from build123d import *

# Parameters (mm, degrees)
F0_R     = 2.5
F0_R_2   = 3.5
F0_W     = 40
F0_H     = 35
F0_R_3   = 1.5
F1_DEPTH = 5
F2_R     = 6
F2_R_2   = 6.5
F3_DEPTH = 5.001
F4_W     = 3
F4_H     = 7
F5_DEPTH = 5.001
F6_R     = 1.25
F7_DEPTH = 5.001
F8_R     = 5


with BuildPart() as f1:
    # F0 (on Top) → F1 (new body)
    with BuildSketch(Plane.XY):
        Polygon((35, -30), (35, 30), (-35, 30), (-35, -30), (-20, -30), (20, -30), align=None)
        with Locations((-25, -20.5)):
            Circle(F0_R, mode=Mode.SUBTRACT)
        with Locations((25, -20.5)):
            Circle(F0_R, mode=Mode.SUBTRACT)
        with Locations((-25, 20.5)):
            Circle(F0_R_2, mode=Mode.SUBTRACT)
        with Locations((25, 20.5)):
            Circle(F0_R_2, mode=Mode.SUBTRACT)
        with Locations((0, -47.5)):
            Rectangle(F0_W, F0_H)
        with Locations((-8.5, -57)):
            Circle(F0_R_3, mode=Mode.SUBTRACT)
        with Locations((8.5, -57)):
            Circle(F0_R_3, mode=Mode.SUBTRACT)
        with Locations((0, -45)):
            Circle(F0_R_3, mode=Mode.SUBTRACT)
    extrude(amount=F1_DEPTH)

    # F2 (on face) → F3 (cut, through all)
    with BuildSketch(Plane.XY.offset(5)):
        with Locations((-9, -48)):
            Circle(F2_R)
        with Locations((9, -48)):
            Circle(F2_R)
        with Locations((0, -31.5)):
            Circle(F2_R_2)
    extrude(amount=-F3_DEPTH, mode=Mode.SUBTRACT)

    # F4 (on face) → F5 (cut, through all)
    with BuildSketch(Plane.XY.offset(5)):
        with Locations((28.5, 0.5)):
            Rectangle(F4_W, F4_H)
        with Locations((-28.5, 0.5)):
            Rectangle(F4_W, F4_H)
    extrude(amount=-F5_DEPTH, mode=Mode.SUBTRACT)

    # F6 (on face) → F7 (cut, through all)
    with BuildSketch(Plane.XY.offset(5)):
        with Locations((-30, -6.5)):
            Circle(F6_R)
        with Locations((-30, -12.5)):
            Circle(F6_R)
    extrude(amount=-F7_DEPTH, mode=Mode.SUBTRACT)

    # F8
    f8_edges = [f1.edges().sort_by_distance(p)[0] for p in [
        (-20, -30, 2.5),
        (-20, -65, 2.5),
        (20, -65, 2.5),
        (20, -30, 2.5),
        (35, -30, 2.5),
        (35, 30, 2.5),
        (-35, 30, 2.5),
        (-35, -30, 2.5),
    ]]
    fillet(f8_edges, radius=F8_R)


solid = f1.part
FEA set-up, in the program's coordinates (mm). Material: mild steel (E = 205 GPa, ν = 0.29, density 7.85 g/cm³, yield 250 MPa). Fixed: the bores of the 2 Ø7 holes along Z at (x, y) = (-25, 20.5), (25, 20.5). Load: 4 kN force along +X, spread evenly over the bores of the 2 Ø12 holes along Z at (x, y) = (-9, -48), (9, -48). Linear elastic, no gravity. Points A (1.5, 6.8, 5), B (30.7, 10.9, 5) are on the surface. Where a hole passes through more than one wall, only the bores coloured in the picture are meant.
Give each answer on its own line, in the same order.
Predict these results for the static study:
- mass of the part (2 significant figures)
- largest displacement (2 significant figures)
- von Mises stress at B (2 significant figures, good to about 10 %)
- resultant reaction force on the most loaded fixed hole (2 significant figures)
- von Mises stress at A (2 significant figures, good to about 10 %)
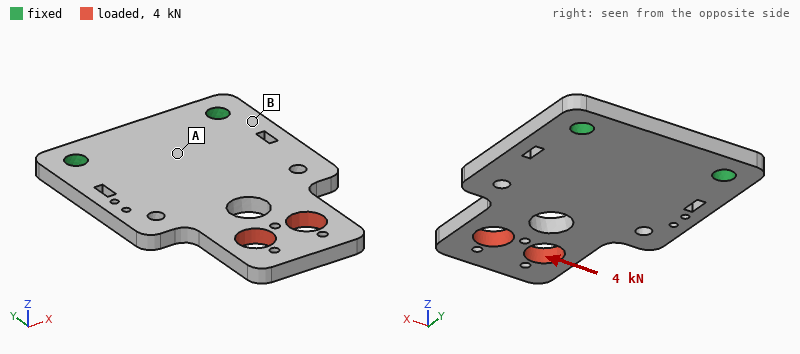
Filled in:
200 g
55 µm
44 MPa
5.5 kN
22 MPa
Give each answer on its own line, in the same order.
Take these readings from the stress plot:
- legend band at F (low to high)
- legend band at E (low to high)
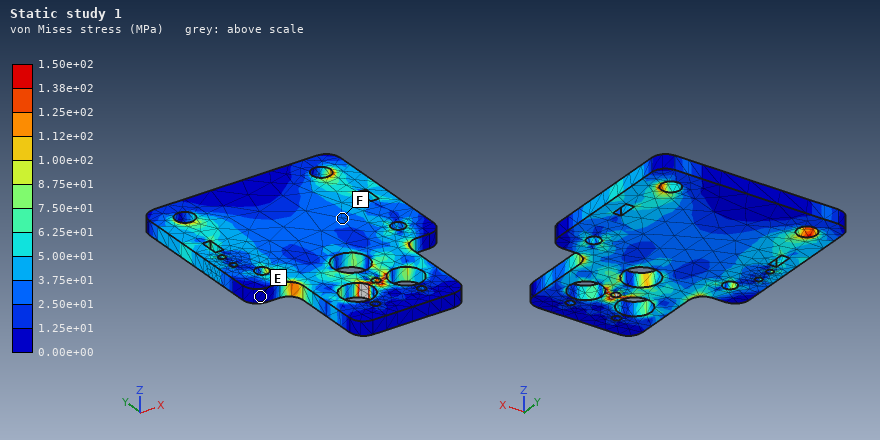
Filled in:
2.50e+01 to 3.75e+01 MPa
0.00e+00 to 1.25e+01 MPa
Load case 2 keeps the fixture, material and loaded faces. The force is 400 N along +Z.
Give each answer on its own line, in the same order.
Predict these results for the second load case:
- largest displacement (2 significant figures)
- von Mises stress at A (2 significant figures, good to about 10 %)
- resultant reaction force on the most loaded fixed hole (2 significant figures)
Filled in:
0.47 mm
63 MPa
200 N
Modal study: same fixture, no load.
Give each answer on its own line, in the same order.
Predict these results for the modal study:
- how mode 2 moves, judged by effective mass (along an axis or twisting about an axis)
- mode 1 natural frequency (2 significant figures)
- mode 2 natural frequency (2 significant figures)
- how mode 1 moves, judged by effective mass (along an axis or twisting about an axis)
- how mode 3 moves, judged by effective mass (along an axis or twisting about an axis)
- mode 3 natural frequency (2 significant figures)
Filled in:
twisting about Y
750 Hz
2600 Hz
along Z
along Z
3100 Hz
